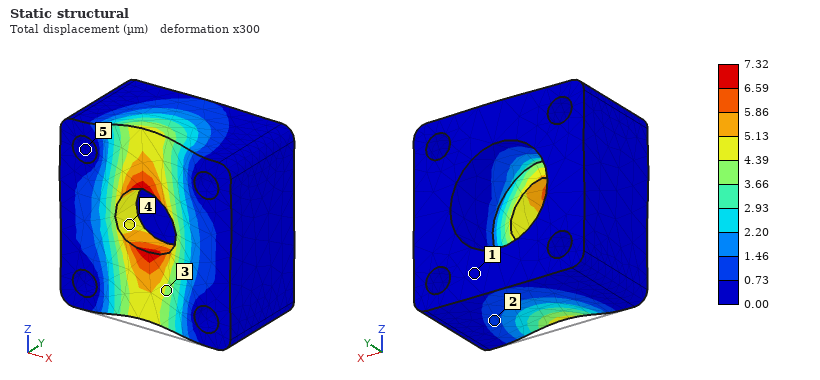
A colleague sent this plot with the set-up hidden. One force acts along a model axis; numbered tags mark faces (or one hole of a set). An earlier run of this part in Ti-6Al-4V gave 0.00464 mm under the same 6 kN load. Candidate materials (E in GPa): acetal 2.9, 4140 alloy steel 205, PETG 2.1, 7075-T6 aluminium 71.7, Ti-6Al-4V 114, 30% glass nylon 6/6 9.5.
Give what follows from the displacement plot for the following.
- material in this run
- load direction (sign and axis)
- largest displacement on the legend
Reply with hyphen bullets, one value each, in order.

- 7075-T6 aluminium
- +Z
- 7.32 µm
